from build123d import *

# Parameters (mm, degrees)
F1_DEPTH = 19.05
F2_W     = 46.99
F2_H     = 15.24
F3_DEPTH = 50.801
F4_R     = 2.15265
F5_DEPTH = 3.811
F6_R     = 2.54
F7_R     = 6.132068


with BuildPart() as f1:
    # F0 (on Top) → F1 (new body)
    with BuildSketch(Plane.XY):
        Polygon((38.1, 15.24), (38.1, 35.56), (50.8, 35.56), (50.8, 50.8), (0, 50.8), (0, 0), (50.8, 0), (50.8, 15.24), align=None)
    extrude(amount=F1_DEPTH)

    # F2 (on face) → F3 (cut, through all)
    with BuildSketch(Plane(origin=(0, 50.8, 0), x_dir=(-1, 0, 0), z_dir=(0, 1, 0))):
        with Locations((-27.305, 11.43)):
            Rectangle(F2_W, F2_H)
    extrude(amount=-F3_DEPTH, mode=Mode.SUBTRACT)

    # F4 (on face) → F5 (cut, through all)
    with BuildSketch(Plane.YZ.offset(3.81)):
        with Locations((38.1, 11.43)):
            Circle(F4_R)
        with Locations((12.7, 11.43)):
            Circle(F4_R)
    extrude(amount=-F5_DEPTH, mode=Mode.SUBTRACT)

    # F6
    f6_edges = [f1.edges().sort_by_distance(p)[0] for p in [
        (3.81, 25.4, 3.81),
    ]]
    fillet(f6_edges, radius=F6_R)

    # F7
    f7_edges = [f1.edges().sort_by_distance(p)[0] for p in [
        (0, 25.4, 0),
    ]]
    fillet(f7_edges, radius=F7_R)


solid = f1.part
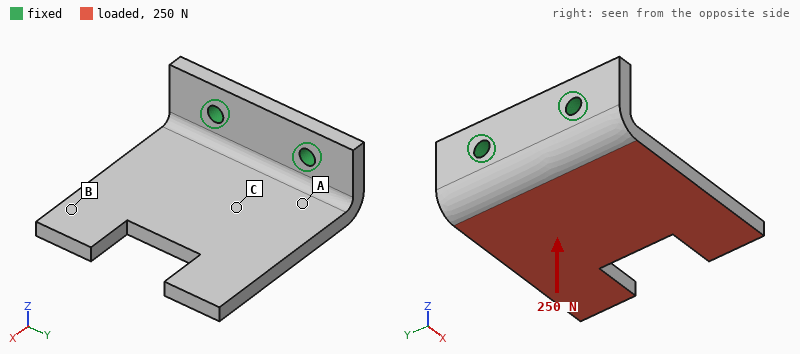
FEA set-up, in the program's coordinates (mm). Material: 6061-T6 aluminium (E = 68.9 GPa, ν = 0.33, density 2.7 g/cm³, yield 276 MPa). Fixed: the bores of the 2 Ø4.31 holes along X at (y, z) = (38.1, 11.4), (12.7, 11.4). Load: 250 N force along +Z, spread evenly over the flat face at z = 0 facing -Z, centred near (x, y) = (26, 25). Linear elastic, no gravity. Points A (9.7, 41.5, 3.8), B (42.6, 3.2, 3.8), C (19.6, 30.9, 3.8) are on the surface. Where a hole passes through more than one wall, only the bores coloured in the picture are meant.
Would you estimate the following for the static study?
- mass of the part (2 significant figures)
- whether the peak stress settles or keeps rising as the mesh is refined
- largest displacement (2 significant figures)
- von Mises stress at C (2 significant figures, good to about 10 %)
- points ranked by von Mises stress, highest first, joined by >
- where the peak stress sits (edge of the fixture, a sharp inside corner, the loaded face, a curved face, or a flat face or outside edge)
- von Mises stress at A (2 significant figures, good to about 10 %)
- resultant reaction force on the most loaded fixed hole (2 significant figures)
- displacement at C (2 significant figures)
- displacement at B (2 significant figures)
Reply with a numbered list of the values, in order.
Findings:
1. 31 g
2. keeps rising
3. 0.35 mm
4. 16 MPa
5. A > C > B
6. edge of the fixture
7. 30 MPa
8. 130 N
9. 0.095 mm
10. 0.28 mm
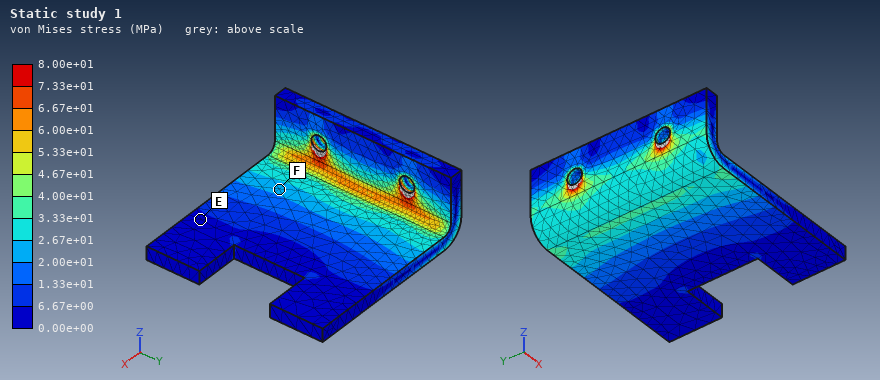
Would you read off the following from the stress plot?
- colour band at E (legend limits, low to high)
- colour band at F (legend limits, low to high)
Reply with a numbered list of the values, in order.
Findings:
1. 0.00e+00 to 6.67e+00 MPa
2. 2.00e+01 to 2.67e+01 MPa
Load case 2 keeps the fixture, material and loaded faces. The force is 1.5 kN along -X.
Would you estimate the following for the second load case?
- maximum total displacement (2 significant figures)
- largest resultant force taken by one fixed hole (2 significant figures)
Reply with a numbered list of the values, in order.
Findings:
1. 0.44 mm
2. 750 N
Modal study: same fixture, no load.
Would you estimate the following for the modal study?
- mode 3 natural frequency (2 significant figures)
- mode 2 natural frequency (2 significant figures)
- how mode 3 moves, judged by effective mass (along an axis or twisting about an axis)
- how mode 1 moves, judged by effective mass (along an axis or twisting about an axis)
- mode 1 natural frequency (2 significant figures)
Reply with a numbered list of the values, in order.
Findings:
1. 4100 Hz
2. 2400 Hz
3. along Y
4. along Z
5. 1200 Hz
